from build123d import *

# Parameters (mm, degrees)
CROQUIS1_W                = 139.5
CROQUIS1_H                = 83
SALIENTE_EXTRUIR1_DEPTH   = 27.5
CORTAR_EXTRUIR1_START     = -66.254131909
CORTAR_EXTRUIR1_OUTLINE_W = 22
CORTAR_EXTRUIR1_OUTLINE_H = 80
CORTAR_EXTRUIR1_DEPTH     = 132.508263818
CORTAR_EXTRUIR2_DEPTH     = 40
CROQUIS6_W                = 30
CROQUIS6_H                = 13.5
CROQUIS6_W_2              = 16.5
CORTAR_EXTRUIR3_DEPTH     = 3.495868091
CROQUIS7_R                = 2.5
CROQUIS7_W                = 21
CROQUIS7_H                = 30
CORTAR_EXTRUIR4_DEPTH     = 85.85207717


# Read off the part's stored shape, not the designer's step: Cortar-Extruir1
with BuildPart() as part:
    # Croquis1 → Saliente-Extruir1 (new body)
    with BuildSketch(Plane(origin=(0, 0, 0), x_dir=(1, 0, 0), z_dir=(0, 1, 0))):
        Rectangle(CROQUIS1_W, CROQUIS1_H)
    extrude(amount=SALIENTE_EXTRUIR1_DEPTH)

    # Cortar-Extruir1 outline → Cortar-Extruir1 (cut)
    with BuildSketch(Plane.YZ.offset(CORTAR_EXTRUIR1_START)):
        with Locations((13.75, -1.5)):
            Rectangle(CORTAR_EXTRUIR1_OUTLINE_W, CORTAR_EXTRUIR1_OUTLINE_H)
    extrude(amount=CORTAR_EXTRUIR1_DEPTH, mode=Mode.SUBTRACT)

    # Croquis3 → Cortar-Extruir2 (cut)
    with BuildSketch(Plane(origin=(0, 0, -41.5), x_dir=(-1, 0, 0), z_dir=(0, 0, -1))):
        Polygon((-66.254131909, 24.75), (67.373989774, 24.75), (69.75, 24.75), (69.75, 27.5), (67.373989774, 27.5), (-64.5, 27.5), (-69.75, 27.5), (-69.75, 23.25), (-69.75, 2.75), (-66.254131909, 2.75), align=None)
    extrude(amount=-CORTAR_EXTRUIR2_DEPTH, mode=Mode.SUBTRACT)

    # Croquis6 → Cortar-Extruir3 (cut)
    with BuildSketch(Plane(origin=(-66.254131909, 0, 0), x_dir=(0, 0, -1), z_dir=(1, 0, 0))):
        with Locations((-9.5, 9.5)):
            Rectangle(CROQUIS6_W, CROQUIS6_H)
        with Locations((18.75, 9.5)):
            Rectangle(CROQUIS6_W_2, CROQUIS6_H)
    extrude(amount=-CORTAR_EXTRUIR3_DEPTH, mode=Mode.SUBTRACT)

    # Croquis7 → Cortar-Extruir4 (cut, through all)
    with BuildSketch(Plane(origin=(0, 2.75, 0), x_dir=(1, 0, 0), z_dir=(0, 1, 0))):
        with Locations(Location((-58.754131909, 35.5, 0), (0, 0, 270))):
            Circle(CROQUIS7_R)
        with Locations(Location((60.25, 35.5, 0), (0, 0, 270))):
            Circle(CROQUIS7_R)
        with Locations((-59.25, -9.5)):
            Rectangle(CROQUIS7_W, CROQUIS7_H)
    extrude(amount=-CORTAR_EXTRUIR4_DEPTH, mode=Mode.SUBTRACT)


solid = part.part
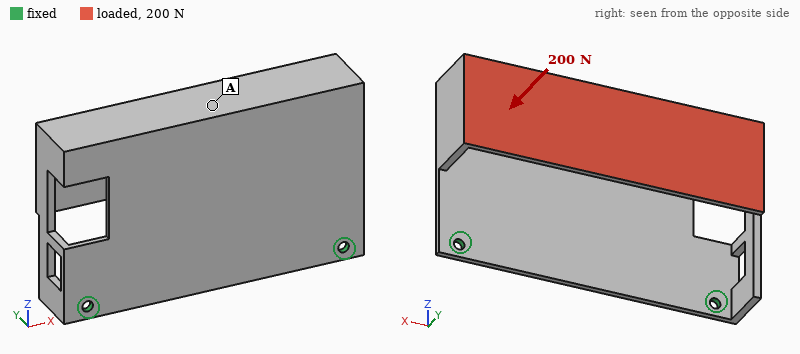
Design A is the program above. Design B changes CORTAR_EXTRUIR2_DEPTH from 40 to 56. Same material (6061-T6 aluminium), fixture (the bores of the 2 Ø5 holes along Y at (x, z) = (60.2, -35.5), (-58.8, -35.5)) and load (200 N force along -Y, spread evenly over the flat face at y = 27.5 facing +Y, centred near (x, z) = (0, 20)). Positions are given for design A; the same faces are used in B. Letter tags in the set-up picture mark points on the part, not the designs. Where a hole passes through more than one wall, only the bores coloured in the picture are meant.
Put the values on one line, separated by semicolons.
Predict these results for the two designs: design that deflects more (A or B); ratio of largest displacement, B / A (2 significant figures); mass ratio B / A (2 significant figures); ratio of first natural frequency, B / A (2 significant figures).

B; 1.3; 0.88; 1.0
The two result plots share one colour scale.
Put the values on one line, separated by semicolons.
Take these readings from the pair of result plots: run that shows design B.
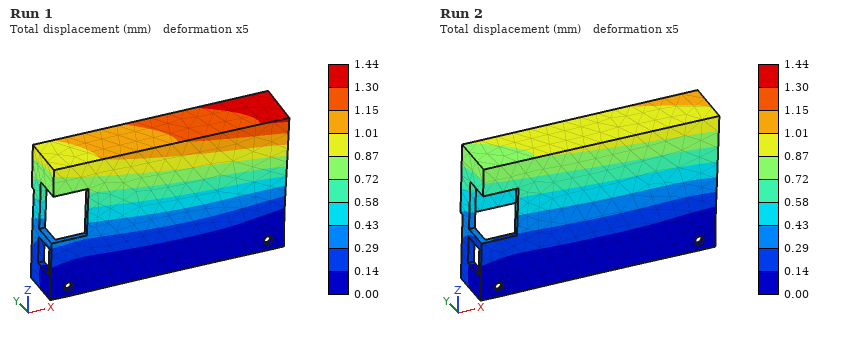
Run 1
